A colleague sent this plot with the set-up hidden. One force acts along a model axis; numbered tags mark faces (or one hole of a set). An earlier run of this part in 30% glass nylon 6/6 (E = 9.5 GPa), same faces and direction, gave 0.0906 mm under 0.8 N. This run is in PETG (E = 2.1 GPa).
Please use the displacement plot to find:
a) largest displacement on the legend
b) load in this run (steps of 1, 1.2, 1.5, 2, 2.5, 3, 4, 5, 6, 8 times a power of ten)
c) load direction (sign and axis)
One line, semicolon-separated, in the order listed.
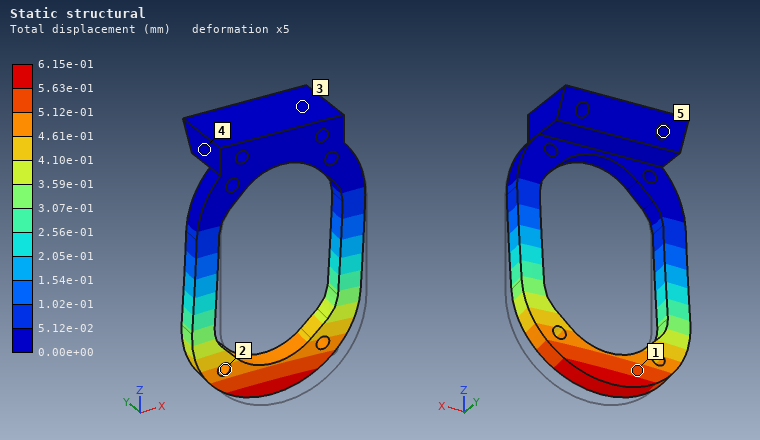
6.15e-01 mm; 1.2 N; +Y
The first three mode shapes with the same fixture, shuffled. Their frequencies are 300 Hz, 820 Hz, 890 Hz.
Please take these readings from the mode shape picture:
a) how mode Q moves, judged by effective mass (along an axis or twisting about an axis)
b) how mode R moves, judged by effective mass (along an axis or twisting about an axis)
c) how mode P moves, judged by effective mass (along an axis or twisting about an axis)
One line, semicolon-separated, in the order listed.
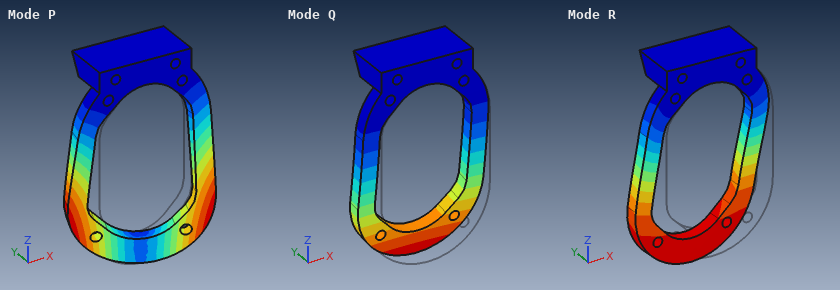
along Y; along X; twisting about Z
